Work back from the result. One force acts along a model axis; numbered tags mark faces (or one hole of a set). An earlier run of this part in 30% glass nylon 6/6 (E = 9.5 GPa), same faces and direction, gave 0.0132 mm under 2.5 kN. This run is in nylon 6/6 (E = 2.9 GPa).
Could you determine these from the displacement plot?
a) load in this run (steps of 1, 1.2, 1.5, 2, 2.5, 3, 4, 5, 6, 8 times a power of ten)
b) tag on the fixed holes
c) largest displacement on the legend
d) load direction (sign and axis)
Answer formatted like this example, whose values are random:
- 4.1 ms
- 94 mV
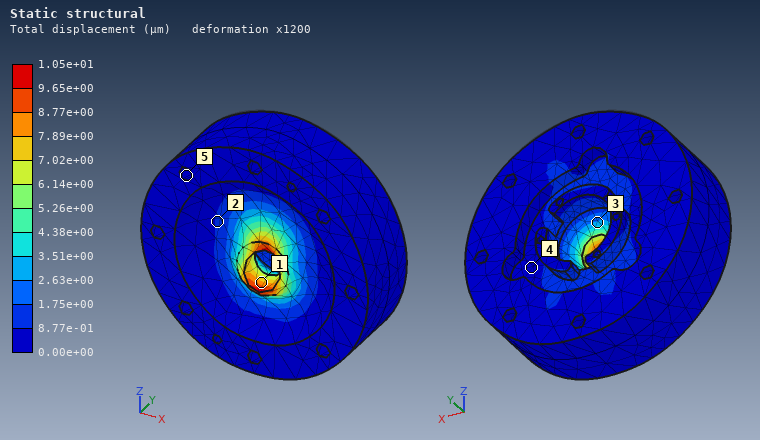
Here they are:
- 600 N
- 5
- 1.05e+01 µm
- -Z
